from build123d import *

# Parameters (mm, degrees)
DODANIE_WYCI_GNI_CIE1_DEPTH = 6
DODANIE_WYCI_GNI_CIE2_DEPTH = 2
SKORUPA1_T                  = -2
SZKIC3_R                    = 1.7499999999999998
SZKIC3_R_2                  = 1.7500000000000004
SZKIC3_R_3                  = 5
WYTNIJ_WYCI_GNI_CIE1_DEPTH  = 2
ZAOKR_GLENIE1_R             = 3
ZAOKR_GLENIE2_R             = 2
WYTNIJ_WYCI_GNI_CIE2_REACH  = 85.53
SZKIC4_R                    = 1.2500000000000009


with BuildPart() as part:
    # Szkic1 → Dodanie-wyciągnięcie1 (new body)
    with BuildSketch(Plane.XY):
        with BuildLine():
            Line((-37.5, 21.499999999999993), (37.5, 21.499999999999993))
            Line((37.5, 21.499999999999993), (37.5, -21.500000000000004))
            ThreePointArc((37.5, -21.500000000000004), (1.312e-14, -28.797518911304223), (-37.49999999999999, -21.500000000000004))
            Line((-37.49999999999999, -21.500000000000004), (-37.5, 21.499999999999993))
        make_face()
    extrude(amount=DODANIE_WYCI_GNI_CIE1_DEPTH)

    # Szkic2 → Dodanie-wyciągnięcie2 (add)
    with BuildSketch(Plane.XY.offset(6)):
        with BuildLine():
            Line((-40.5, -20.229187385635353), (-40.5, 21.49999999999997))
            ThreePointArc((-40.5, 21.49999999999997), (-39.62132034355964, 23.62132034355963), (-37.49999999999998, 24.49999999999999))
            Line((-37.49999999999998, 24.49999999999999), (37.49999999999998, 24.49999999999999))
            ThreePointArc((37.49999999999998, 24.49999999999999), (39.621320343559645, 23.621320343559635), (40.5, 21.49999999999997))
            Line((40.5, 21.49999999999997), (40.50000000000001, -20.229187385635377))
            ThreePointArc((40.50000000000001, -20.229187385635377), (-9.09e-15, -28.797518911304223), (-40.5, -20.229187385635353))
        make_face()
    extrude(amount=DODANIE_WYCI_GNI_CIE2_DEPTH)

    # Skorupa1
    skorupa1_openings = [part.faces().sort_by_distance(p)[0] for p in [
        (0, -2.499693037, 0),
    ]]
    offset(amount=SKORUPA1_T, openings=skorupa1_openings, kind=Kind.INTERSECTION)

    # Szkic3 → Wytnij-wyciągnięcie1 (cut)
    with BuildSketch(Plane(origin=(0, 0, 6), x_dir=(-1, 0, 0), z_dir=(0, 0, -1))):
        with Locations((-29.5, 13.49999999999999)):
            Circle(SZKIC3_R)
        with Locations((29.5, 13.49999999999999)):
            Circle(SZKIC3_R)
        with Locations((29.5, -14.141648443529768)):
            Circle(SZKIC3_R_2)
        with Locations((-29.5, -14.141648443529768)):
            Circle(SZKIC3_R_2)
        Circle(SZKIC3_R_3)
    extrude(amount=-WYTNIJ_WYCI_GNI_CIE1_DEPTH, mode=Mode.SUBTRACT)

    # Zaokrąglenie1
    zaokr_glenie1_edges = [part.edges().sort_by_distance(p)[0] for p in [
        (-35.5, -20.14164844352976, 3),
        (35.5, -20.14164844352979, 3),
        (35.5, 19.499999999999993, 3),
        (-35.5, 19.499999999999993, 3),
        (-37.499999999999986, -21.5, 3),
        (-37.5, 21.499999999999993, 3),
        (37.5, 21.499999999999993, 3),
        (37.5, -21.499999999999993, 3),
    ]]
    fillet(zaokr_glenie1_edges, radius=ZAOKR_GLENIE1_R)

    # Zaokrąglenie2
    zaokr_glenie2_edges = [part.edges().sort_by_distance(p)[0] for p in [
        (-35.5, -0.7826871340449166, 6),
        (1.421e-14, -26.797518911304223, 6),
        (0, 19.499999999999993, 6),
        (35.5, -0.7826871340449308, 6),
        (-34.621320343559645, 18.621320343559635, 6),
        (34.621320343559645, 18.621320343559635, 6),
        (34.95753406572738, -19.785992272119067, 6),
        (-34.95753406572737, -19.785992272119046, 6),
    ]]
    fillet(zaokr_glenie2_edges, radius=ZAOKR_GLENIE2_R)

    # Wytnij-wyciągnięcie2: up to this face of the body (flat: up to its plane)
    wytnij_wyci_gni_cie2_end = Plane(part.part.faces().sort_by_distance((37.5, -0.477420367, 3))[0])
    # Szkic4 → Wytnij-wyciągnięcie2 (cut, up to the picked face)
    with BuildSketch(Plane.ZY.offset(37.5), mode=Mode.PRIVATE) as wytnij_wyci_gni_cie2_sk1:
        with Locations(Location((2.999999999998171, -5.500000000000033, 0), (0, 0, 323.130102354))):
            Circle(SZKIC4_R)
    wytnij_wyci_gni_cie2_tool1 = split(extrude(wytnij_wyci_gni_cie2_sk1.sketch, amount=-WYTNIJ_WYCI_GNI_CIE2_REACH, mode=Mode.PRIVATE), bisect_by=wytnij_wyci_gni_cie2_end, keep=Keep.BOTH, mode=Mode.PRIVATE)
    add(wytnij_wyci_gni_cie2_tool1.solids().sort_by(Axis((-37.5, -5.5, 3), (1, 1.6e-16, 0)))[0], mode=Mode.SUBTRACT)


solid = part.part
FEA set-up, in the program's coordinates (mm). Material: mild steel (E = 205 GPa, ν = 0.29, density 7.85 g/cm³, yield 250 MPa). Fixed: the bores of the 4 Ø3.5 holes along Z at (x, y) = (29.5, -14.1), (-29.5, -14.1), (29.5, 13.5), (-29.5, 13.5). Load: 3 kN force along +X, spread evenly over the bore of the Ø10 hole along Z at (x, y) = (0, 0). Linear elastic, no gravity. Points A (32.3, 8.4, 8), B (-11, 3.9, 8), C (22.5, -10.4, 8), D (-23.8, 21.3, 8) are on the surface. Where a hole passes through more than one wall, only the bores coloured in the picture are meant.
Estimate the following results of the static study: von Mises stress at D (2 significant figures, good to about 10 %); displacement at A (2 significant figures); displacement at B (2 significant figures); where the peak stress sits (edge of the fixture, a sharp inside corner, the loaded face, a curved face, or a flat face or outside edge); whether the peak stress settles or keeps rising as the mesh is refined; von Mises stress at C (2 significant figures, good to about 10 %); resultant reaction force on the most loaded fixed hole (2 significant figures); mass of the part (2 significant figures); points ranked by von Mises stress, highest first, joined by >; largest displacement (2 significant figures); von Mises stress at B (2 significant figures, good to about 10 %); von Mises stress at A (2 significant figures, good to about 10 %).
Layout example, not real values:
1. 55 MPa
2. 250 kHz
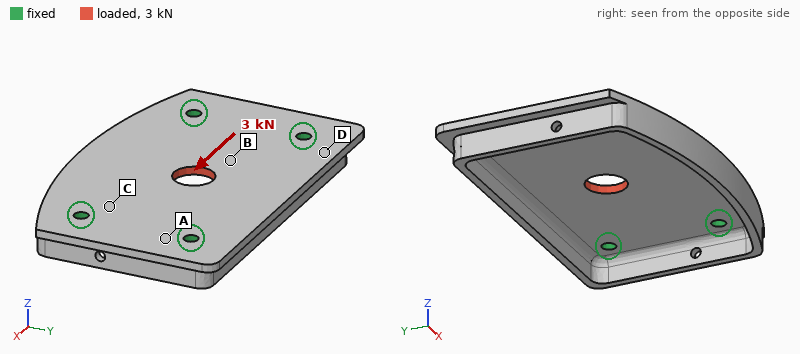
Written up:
1. 7.0 MPa
2. 0.66 µm
3. 2.8 µm
4. a sharp inside corner
5. keeps rising
6. 26 MPa
7. 780 N
8. 85 g
9. B > C > A > D
10. 4.3 µm
11. 34 MPa
12. 16 MPa
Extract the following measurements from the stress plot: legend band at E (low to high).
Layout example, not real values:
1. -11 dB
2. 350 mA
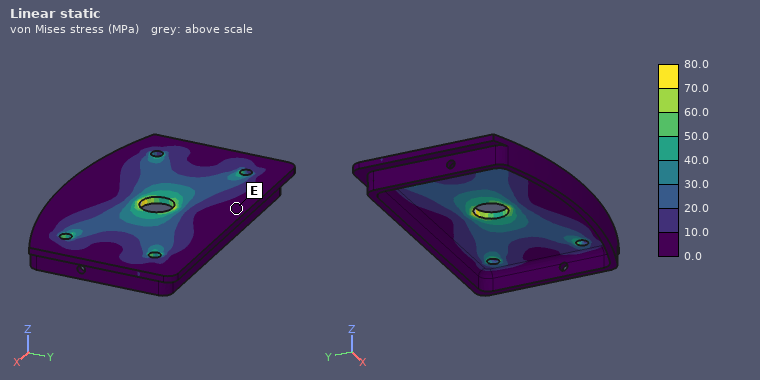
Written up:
1. 0.0 to 10.0 MPa
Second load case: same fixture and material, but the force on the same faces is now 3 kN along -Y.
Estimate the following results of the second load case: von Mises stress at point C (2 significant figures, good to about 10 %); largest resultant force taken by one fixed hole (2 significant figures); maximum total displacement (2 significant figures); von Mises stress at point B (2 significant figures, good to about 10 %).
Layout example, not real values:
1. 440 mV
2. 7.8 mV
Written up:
1. 31 MPa
2. 860 N
3. 9.3 µm
4. 31 MPa
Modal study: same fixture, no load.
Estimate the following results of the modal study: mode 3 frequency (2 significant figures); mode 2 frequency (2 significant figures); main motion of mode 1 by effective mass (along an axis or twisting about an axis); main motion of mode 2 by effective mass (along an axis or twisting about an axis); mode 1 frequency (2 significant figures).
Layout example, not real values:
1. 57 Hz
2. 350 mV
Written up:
1. 6000 Hz
2. 4900 Hz
3. along Z
4. twisting about X
5. 4100 Hz
